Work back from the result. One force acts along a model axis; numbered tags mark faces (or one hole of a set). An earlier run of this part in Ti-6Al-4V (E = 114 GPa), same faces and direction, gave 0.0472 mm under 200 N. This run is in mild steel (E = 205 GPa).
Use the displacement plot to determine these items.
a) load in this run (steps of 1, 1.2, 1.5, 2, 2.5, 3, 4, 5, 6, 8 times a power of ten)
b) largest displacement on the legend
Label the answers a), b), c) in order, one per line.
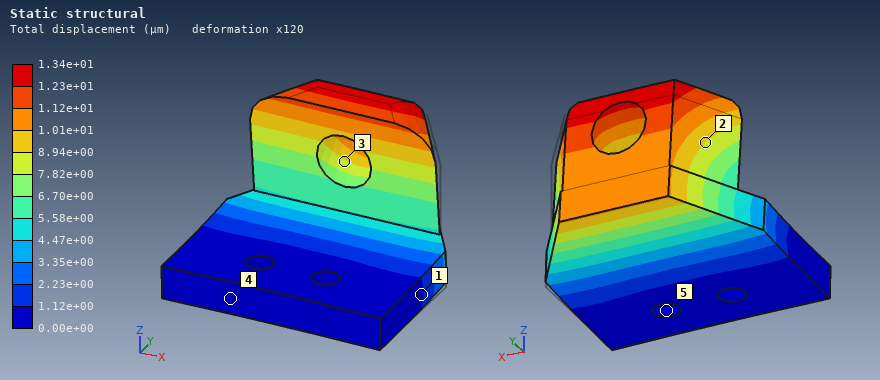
a) 100 N
b) 1.34e+01 µm
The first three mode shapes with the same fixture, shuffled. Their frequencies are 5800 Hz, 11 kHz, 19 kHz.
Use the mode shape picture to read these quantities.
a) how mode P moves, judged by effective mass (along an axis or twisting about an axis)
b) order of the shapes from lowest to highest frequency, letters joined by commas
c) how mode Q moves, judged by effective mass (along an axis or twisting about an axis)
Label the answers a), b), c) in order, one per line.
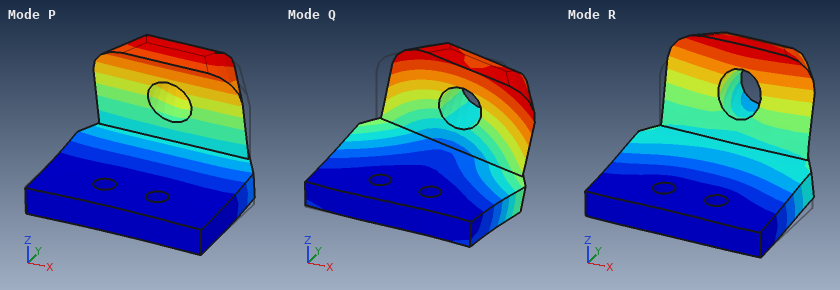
a) along Z
b) P, Q, R
c) along X
